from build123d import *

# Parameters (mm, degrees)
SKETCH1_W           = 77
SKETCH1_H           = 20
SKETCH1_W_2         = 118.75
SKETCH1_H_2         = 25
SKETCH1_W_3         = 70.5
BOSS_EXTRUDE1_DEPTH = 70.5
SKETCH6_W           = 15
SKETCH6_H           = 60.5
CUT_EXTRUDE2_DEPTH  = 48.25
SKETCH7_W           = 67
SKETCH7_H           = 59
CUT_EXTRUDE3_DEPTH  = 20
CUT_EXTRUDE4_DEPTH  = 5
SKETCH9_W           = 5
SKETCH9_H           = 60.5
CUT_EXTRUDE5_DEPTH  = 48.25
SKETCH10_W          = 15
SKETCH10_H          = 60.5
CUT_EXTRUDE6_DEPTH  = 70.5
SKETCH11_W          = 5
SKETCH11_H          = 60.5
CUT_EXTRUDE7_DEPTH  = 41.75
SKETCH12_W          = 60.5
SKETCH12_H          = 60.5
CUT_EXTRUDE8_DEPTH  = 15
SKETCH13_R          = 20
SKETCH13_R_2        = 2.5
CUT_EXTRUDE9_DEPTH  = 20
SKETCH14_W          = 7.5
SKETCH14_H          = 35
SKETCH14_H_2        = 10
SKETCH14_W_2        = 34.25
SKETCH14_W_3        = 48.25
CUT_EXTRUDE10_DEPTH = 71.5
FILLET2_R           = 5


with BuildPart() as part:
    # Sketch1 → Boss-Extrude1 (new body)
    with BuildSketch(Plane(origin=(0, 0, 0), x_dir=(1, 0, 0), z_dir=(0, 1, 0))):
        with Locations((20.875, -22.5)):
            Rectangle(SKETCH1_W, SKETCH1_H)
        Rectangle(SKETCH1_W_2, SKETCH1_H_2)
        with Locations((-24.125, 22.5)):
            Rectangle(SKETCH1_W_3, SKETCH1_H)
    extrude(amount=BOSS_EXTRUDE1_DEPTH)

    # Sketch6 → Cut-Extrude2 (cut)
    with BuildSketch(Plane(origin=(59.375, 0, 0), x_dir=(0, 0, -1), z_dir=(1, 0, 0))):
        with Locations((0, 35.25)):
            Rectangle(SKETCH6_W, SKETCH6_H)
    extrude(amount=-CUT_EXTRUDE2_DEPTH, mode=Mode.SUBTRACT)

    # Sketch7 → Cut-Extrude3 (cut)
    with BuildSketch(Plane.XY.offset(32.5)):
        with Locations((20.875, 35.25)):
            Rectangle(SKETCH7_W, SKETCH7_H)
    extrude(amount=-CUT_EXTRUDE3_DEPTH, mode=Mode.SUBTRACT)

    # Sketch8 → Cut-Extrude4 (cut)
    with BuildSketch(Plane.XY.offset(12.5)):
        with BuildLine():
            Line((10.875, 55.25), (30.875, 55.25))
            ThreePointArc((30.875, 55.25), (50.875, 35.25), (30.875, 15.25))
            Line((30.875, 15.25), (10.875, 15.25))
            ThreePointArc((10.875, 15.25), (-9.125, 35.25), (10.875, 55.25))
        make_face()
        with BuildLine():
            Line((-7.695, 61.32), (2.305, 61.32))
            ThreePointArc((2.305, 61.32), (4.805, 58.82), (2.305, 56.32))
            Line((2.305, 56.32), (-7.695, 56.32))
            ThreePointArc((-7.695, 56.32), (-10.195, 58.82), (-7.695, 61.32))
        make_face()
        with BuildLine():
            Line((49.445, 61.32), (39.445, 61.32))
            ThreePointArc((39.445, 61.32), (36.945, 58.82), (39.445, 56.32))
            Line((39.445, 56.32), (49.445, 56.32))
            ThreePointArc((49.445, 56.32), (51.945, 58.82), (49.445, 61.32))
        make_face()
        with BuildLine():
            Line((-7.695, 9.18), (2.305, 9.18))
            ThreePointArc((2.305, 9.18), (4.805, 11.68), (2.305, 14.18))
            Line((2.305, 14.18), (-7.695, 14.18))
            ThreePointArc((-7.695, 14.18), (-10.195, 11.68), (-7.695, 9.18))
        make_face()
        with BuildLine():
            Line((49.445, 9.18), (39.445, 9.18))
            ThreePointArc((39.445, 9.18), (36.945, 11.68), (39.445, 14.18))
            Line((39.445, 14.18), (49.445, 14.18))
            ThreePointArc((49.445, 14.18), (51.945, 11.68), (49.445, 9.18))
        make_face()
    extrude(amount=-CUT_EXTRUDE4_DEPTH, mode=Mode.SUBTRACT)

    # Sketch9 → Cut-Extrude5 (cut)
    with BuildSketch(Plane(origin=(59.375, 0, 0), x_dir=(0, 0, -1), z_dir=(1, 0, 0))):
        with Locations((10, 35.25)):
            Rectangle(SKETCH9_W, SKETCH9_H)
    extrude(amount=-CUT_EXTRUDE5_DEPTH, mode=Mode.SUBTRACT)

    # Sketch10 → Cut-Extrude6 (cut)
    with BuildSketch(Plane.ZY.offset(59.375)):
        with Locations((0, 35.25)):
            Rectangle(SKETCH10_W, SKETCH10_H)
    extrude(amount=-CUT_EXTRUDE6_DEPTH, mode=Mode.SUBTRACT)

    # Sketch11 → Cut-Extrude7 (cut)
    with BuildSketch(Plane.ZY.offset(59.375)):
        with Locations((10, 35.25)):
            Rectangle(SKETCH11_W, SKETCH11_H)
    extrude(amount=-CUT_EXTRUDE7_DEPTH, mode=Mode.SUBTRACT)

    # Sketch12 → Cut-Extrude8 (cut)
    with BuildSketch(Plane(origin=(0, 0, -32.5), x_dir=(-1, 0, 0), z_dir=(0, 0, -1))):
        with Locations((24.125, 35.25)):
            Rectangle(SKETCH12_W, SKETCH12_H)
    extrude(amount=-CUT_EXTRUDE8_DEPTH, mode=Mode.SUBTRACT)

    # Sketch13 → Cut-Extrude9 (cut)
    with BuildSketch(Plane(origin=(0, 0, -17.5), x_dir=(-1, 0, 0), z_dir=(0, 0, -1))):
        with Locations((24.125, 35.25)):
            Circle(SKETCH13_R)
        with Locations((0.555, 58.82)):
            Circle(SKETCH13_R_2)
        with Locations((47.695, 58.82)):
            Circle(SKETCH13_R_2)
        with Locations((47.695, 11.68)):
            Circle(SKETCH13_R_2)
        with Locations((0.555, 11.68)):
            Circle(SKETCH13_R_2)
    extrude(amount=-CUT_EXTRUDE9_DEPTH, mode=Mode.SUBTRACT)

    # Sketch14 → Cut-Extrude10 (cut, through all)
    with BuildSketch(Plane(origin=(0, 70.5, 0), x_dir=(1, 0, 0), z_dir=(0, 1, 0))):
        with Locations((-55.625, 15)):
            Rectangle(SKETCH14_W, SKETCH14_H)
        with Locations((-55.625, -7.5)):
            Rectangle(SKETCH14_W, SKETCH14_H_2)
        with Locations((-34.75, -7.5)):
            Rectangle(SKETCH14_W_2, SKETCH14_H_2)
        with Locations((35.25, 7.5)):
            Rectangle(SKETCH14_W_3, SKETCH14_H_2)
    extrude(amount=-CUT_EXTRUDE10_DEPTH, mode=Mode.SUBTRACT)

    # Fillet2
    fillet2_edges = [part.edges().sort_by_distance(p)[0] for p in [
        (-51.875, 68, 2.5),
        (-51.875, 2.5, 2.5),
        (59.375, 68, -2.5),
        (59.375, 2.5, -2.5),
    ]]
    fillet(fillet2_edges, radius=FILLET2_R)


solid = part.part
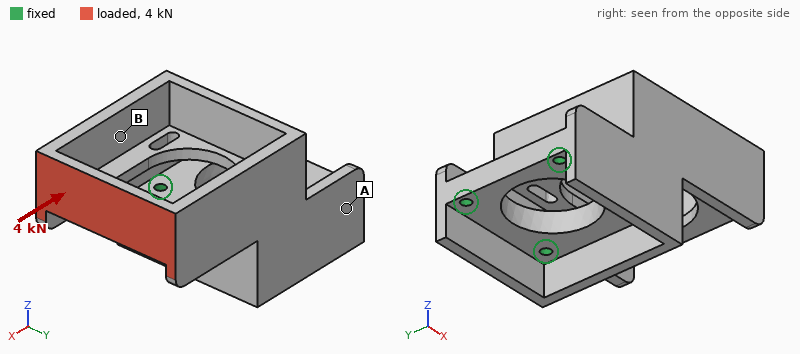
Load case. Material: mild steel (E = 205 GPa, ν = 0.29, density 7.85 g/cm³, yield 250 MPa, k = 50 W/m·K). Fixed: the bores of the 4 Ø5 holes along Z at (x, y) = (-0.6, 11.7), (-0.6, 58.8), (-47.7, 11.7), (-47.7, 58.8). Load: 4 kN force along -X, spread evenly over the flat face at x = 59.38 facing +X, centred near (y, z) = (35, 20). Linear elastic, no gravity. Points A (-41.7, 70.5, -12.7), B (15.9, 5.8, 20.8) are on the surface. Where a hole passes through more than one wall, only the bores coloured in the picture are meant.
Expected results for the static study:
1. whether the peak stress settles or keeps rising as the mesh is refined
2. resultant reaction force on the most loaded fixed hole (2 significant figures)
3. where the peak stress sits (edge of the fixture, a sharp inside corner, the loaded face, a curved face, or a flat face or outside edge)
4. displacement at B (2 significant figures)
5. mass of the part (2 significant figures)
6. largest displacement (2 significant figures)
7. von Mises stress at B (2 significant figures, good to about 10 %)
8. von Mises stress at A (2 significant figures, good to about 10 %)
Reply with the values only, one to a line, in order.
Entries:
keeps rising
1.7 kN
edge of the fixture
21 µm
800 g
82 µm
16 MPa
9.6 MPa
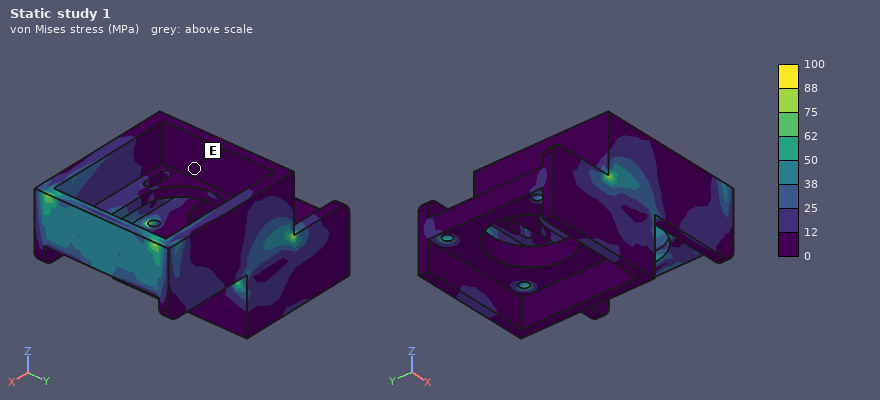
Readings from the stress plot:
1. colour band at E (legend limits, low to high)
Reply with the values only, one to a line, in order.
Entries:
0 to 12 MPa
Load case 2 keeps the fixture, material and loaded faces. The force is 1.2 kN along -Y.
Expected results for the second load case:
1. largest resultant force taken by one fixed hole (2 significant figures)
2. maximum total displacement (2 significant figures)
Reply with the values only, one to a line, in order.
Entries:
1.1 kN
48 µm
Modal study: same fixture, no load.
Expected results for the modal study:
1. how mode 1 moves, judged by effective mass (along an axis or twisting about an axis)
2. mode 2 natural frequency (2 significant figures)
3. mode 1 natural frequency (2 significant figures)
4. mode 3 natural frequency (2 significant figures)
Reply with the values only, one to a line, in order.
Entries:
along Y
2200 Hz
1900 Hz
3100 Hz
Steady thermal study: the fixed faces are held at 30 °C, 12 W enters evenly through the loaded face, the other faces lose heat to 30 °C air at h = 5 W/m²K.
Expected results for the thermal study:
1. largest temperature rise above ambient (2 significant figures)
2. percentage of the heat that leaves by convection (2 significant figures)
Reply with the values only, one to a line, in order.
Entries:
46 K
21 %
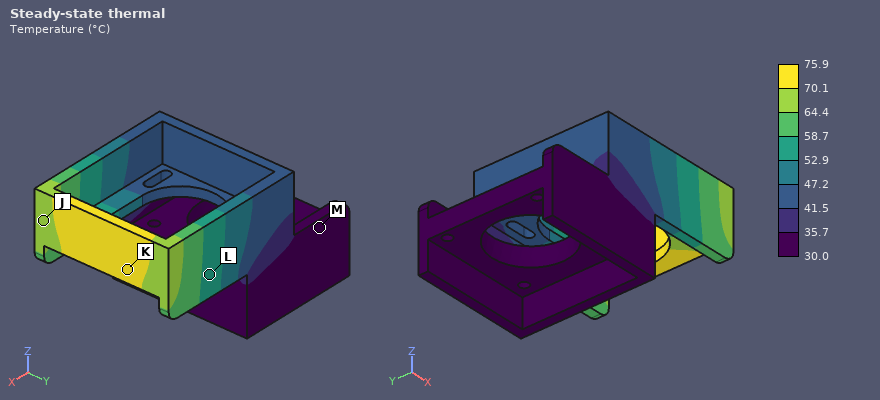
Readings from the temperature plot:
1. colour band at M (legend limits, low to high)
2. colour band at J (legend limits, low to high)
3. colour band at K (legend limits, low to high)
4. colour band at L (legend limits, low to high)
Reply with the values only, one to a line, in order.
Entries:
30.0 to 35.7 °C
64.4 to 70.1 °C
70.1 to 75.9 °C
52.9 to 58.7 °C
